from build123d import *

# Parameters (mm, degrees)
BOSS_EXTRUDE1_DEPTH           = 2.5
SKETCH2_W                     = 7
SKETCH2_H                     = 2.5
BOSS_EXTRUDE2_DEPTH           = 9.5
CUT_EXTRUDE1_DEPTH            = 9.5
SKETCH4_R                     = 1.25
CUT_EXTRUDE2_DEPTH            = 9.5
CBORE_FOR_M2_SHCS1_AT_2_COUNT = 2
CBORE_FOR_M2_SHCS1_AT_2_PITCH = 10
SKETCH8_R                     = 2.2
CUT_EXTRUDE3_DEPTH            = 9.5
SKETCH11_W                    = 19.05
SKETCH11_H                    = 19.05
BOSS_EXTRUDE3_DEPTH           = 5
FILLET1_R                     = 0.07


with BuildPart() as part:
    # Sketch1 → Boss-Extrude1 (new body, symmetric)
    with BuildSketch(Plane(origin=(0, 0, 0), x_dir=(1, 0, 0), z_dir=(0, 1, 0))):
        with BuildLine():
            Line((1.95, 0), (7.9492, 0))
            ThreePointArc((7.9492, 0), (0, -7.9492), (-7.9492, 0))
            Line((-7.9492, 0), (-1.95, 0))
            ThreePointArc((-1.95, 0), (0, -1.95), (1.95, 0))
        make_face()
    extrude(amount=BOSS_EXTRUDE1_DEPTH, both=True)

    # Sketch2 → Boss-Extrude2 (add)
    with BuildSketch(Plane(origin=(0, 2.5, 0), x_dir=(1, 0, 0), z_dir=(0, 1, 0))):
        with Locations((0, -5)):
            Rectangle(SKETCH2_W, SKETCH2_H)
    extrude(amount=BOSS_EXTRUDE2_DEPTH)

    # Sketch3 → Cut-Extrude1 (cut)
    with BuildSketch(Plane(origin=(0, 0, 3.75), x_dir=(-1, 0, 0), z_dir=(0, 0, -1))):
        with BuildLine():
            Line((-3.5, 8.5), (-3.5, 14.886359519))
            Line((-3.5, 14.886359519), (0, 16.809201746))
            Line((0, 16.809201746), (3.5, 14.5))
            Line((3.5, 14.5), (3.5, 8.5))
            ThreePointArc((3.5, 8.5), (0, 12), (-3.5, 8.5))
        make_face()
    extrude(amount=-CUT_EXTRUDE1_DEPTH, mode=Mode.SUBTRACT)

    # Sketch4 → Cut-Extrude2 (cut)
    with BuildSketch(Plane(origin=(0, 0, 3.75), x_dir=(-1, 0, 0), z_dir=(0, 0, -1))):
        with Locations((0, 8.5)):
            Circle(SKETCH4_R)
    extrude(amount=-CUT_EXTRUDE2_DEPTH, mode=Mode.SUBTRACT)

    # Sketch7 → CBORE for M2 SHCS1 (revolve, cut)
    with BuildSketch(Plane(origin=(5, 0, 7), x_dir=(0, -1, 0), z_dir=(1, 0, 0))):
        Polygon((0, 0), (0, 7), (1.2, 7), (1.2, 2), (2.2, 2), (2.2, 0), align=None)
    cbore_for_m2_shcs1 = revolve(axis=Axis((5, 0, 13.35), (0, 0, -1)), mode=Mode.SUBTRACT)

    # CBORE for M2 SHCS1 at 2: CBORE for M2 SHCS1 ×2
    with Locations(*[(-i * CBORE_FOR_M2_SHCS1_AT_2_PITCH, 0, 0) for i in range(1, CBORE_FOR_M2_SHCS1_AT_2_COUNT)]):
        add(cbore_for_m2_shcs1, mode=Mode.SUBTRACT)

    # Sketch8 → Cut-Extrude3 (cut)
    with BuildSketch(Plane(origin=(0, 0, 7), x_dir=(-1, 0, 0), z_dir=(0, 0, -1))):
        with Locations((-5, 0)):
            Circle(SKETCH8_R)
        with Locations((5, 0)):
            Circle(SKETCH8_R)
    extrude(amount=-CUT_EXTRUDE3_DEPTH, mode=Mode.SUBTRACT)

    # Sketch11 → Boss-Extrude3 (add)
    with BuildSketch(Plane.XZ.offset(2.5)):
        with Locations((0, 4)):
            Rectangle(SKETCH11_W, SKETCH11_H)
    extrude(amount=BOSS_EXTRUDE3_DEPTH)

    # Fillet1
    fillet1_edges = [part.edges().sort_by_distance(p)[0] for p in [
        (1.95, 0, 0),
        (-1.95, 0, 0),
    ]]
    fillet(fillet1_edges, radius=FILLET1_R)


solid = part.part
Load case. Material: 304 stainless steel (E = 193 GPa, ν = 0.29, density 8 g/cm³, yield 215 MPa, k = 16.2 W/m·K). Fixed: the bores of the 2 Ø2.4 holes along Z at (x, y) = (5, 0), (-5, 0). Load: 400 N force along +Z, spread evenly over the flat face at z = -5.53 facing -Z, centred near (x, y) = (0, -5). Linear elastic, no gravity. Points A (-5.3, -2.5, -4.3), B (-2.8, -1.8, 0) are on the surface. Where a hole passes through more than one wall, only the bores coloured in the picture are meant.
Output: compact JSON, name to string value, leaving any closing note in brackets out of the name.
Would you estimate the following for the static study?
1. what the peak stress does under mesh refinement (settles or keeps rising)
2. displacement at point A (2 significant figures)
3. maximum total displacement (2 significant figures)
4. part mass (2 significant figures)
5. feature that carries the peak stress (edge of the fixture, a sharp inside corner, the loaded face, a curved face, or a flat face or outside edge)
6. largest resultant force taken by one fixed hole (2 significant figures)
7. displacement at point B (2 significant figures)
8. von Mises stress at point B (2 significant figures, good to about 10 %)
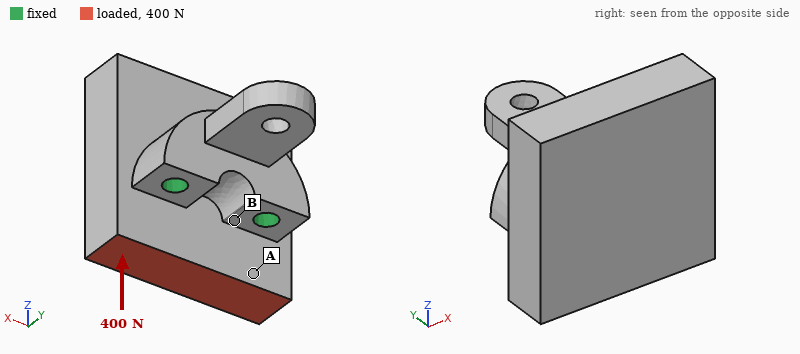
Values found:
{"what the peak stress does under mesh refinement": "keeps rising", "displacement at point A": "1.2 µm", "maximum total displacement": "2.1 µm", "part mass": "19 g", "feature that carries the peak stress": "edge of the fixture", "largest resultant force taken by one fixed hole": "200 N", "displacement at point B": "0.40 µm", "von Mises stress at point B": "15 MPa"}
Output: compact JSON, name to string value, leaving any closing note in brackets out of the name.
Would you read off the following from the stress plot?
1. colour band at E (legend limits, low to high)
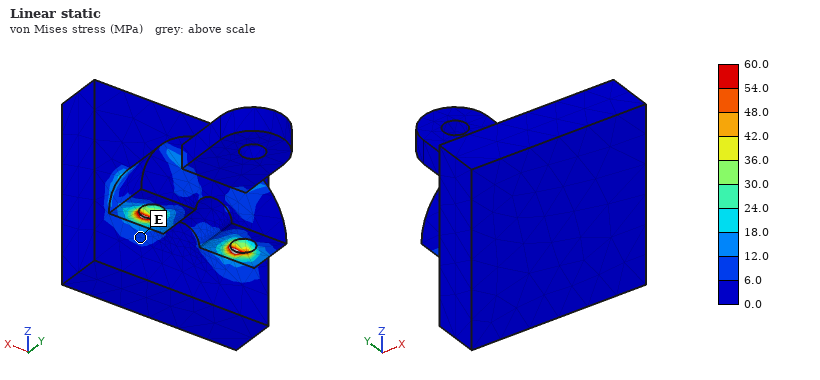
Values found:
{"colour band at E": "6.0 to 12.0 MPa"}
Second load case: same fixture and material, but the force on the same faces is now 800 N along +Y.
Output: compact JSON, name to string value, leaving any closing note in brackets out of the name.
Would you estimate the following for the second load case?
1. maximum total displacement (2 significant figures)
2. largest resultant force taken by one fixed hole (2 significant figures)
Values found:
{"maximum total displacement": "11 µm", "largest resultant force taken by one fixed hole": "400 N"}
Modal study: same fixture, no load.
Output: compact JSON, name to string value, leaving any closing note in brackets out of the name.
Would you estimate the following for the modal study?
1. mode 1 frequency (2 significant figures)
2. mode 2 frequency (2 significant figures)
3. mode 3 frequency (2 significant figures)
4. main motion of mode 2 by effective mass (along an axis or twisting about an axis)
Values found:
{"mode 1 frequency": "17 kHz", "mode 2 frequency": "22 kHz", "mode 3 frequency": "29 kHz", "main motion of mode 2 by effective mass": "along Z"}
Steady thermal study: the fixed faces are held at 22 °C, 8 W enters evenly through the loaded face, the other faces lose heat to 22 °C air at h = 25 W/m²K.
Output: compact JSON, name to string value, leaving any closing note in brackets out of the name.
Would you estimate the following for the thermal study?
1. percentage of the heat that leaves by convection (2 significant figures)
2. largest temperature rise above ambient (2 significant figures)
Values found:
{"percentage of the heat that leaves by convection": "8.1 %", "largest temperature rise above ambient": "57 K"}
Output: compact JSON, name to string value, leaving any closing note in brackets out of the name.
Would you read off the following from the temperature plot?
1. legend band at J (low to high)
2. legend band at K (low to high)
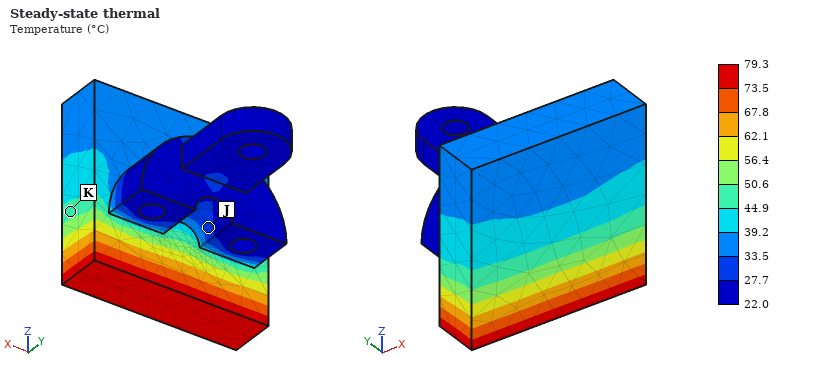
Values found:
{"legend band at J": "27.7 to 33.5 °C", "legend band at K": "44.9 to 50.6 °C"}
